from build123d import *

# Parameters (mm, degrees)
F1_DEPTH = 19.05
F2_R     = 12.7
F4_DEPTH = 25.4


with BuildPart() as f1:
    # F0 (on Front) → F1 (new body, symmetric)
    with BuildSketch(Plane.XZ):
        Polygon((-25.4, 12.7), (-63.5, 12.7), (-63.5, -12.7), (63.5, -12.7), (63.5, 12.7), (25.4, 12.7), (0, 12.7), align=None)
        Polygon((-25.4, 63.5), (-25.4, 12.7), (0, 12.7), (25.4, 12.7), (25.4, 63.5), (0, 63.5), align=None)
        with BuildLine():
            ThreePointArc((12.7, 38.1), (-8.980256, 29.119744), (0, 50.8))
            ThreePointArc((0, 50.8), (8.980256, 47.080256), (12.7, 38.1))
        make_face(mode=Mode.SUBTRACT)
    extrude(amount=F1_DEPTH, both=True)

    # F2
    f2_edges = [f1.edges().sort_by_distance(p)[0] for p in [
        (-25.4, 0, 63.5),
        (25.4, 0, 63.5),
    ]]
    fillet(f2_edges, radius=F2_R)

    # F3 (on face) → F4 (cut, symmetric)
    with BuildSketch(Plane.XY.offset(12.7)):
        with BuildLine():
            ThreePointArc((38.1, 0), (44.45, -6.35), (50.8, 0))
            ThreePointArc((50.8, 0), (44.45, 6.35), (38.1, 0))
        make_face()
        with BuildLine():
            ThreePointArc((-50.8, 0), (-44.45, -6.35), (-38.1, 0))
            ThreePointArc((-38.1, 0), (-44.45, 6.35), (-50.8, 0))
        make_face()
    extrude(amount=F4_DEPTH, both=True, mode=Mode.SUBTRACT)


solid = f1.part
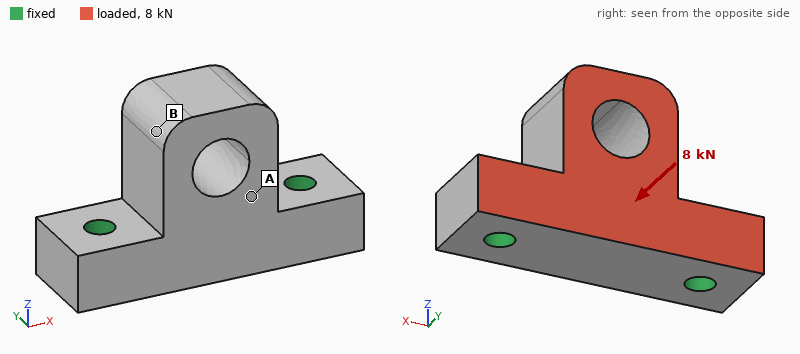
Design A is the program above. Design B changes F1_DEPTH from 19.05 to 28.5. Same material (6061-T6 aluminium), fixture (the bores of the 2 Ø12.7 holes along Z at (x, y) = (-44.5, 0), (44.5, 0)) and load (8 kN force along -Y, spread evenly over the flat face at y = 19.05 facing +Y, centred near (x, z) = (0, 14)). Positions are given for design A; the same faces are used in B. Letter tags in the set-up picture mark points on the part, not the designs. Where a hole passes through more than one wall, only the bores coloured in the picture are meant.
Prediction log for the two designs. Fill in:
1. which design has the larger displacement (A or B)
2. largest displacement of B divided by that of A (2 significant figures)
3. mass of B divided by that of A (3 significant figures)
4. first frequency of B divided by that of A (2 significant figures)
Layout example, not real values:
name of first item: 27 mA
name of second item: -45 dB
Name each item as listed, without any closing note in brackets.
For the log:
which design has the larger displacement: A
largest displacement of B divided by that of A: 0.59
mass of B divided by that of A: 1.51
first frequency of B divided by that of A: 1.0
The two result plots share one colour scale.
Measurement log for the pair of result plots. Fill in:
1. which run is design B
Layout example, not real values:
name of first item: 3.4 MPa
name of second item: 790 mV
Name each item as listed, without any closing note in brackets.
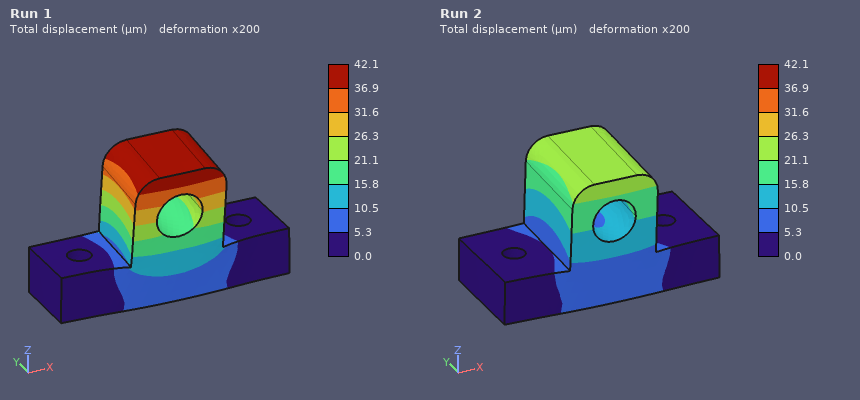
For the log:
which run is design B: Run 2
